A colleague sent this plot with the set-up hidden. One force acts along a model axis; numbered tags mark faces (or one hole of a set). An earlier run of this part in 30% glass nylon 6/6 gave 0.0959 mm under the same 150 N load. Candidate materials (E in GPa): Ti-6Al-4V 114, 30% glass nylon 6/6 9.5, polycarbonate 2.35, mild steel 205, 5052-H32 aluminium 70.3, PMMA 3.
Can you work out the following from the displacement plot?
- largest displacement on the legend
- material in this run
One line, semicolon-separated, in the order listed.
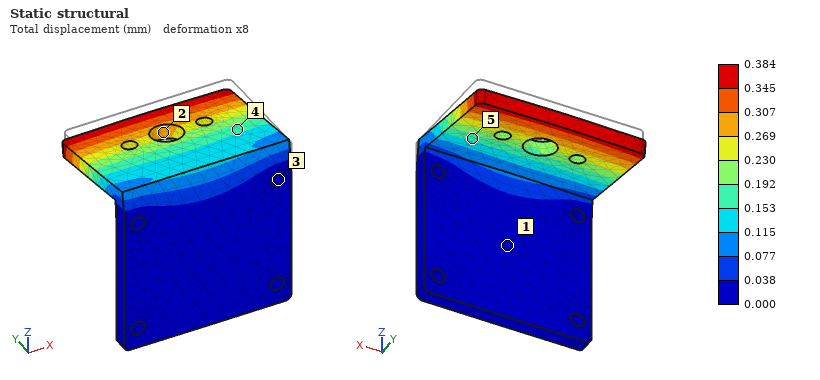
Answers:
0.384 mm; polycarbonate
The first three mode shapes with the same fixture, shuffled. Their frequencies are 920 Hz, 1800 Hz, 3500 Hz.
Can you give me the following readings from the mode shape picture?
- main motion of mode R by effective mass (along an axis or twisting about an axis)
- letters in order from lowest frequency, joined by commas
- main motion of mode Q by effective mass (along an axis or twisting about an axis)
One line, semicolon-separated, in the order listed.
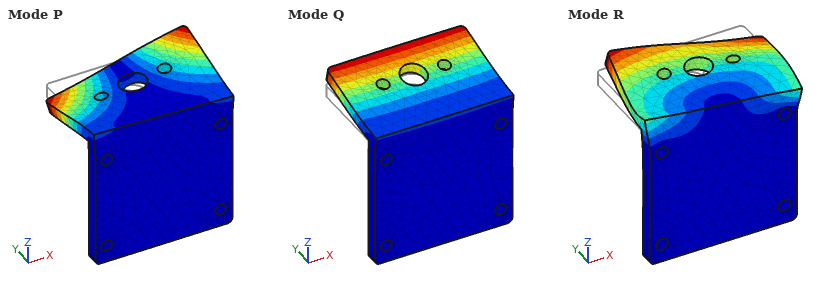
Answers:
along X; Q, P, R; along Z
